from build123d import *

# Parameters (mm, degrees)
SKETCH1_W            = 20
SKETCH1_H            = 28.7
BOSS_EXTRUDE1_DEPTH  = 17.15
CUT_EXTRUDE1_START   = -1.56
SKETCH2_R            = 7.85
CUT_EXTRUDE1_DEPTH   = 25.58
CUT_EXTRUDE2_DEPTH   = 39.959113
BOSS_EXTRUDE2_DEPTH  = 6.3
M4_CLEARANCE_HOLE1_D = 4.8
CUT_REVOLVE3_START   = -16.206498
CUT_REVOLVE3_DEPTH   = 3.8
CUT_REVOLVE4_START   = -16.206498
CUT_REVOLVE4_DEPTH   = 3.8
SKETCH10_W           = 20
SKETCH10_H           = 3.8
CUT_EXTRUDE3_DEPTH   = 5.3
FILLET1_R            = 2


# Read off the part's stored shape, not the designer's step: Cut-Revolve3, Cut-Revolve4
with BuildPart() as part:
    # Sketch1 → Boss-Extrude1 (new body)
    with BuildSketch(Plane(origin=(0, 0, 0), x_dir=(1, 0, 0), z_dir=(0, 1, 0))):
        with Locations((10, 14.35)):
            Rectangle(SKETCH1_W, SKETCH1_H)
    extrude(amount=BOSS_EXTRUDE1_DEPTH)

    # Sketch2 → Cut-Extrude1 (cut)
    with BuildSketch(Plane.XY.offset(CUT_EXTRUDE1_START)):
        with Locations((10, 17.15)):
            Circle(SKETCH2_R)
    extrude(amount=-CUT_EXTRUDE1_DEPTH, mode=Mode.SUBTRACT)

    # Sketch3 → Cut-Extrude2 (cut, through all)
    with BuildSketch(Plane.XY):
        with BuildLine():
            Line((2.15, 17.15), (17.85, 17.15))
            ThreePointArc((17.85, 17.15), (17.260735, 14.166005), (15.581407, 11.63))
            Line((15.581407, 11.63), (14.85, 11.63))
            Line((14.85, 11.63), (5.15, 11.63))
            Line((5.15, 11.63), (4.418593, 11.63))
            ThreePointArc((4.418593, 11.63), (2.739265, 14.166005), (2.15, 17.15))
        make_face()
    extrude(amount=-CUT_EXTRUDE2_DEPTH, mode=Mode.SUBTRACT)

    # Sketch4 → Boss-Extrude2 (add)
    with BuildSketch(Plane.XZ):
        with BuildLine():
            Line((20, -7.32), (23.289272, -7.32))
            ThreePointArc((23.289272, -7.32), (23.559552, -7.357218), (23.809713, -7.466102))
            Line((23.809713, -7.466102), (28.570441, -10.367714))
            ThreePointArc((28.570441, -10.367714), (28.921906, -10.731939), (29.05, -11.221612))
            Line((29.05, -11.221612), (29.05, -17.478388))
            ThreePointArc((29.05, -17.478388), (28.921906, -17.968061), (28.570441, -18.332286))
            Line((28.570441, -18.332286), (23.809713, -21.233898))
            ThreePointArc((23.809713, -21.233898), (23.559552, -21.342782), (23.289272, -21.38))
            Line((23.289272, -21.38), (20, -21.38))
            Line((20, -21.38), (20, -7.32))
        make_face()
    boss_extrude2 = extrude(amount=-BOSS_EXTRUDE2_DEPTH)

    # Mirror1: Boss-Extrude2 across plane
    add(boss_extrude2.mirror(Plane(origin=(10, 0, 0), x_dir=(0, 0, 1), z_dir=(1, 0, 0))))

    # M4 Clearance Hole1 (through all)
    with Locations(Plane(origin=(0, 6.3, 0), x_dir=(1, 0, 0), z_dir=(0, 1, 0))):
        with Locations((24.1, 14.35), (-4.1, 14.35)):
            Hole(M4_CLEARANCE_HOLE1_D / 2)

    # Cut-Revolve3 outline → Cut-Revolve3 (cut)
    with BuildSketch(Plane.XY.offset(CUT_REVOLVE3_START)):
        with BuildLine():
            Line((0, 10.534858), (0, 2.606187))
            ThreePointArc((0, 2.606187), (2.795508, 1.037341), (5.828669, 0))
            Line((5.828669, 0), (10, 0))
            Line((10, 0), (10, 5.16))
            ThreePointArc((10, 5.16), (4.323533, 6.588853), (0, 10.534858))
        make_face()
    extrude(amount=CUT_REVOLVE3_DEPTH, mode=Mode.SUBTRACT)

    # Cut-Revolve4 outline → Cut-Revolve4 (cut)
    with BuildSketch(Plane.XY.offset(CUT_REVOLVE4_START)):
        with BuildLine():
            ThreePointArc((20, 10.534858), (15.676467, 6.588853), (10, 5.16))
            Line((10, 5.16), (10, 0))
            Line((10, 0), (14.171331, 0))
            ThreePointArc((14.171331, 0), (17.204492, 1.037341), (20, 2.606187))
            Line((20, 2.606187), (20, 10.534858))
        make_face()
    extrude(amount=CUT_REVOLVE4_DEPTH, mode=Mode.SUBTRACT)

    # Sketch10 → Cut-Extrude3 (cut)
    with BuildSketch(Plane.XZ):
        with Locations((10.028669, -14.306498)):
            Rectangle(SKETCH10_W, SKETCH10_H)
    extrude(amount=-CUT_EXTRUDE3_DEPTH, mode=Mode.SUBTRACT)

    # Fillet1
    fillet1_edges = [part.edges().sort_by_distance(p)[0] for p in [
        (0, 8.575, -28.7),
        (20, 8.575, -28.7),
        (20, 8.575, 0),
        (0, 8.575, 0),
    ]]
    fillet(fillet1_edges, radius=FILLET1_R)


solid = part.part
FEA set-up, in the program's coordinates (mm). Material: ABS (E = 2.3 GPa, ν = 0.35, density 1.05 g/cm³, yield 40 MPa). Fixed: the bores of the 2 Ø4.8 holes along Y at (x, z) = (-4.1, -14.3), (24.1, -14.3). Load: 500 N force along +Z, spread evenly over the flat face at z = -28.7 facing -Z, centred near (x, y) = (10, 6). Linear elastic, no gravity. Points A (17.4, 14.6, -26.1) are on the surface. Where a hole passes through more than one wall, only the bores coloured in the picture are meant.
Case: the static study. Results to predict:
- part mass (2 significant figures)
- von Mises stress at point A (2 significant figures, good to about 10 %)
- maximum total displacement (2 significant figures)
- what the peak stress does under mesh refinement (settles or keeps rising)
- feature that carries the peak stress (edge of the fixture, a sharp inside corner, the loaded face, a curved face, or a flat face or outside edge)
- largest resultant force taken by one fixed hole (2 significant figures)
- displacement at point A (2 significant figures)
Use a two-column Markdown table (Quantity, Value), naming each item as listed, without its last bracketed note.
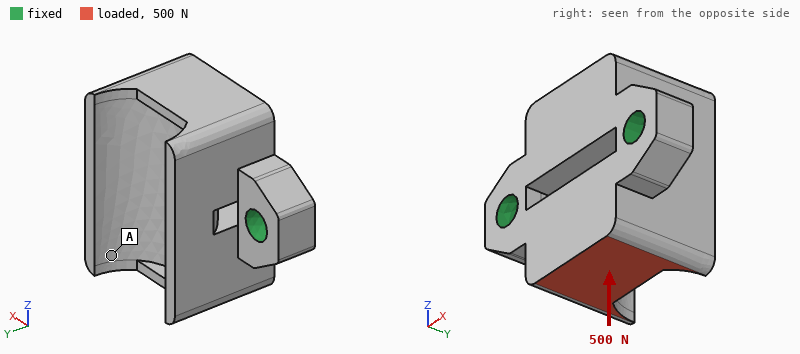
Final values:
| Quantity | Value |
|---|---|
| part mass | 8.1 g |
| von Mises stress at point A | 2.1 MPa |
| maximum total displacement | 0.16 mm |
| what the peak stress does under mesh refinement | keeps rising |
| feature that carries the peak stress | a sharp inside corner |
| largest resultant force taken by one fixed hole | 260 N |
| displacement at point A | 0.12 mm |
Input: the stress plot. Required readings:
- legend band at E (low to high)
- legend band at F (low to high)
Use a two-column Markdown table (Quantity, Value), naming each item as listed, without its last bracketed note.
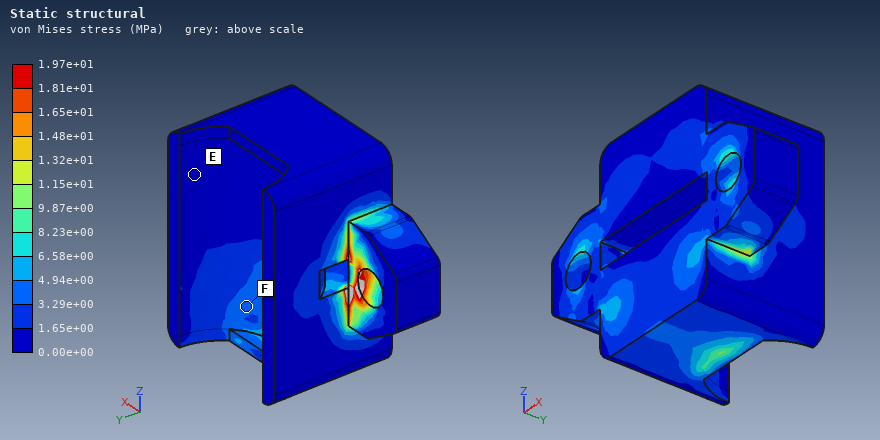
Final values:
| Quantity | Value |
|---|---|
| legend band at E | 0.00e+00 to 1.65e+00 MPa |
| legend band at F | 3.29e+00 to 4.94e+00 MPa |
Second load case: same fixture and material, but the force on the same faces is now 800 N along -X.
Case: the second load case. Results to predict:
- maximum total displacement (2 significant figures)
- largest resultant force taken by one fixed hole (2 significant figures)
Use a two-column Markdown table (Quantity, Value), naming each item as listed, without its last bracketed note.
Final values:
| Quantity | Value |
|---|---|
| maximum total displacement | 0.16 mm |
| largest resultant force taken by one fixed hole | 570 N |
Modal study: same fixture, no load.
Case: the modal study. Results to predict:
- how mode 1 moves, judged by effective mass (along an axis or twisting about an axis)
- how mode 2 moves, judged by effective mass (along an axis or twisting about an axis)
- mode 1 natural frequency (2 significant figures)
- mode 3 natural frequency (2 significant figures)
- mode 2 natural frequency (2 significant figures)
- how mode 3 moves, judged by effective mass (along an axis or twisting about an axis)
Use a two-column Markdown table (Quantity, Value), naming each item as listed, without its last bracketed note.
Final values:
| Quantity | Value |
|---|---|
| how mode 1 moves, judged by effective mass | along Z |
| how mode 2 moves, judged by effective mass | along Y |
| mode 1 natural frequency | 3100 Hz |
| mode 3 natural frequency | 8300 Hz |
| mode 2 natural frequency | 6000 Hz |
| how mode 3 moves, judged by effective mass | along X |
